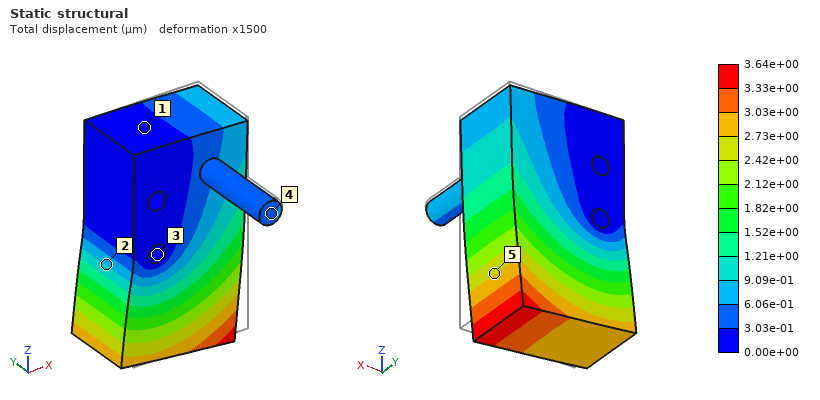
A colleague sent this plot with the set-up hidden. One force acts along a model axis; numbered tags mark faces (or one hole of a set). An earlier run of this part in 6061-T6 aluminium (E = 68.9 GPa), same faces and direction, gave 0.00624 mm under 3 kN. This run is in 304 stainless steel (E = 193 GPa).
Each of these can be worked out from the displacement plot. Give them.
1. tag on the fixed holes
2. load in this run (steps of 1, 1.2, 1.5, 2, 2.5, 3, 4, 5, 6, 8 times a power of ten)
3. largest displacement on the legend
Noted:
3
5 kN
3.64e+00 µm
